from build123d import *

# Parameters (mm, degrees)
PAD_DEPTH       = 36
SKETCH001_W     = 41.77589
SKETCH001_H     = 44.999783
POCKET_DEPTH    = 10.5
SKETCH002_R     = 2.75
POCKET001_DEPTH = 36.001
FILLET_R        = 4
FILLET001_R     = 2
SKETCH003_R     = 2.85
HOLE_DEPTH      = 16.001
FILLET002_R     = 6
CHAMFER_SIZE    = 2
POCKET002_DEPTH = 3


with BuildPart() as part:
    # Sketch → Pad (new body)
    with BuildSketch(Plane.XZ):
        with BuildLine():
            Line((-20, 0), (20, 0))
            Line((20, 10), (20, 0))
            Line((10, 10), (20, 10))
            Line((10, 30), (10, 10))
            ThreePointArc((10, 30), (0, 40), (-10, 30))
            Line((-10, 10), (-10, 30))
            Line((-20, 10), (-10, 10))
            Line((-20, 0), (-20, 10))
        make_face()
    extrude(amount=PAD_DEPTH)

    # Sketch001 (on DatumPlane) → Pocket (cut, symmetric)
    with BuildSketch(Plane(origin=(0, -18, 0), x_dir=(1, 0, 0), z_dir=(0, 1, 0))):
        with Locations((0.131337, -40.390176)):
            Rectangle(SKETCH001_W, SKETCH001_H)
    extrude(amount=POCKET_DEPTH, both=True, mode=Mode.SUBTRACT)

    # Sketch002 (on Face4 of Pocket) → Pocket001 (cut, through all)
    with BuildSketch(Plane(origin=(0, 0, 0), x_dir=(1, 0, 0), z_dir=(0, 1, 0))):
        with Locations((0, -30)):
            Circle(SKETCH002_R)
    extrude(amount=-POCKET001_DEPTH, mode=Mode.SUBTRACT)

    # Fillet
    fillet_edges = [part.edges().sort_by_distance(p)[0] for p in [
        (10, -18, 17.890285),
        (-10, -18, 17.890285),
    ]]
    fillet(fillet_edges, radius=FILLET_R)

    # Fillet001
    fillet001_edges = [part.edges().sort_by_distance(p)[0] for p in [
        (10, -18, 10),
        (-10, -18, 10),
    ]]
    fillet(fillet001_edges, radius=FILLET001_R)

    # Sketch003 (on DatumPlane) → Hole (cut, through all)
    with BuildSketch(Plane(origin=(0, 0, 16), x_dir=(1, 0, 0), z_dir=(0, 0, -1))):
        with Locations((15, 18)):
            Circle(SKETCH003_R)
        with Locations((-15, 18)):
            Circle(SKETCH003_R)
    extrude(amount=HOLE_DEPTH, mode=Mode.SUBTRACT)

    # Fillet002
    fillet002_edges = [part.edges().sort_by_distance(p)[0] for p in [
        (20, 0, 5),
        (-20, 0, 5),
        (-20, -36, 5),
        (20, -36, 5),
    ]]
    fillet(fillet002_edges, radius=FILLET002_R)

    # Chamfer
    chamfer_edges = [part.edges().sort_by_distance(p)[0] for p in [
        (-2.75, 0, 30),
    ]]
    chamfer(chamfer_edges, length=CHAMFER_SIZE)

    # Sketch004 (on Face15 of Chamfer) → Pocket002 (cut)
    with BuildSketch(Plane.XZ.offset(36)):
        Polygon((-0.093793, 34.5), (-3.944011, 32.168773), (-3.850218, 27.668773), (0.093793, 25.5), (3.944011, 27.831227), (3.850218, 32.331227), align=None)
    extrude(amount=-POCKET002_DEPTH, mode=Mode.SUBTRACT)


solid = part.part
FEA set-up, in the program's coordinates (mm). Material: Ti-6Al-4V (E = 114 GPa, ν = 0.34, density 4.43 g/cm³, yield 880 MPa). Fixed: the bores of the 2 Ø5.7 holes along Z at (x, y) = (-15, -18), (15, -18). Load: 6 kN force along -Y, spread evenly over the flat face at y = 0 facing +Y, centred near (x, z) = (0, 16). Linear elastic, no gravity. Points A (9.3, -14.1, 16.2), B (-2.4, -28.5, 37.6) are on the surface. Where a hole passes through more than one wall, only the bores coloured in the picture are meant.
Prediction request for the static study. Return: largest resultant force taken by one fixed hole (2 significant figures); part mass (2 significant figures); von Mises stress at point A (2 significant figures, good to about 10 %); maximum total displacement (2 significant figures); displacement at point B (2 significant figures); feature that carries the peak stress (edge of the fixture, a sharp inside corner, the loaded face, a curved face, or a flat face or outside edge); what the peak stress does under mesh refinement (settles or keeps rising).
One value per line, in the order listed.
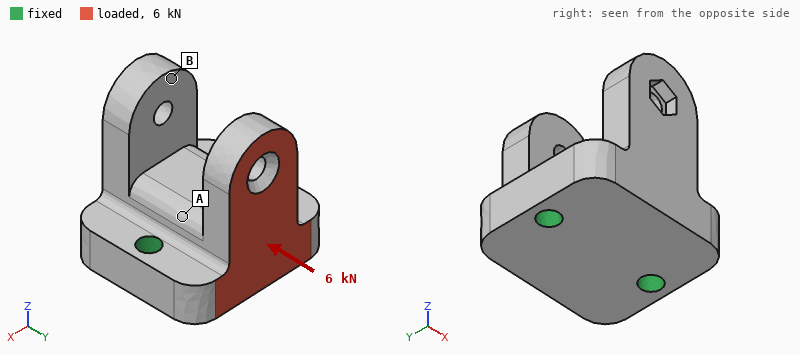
3.0 kN
110 g
37 MPa
0.13 mm
0.029 mm
edge of the fixture
keeps rising
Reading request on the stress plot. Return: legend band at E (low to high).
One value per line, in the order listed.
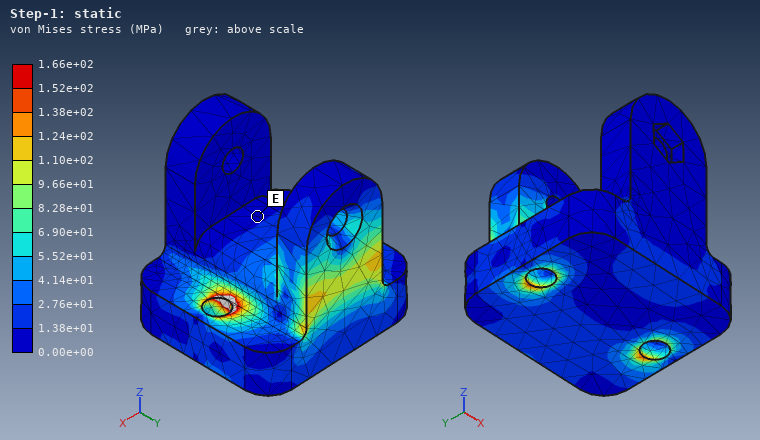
0.00e+00 to 1.38e+01 MPa
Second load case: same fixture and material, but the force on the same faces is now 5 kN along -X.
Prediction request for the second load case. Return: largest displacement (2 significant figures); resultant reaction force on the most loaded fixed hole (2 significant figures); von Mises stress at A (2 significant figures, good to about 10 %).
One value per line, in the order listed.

39 µm
4.2 kN
22 MPa
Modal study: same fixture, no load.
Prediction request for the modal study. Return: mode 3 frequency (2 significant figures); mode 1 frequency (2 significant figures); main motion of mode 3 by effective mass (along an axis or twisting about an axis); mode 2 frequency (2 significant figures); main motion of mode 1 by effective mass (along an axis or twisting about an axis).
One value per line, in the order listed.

13 kHz
6900 Hz
along X
9500 Hz
along Y
